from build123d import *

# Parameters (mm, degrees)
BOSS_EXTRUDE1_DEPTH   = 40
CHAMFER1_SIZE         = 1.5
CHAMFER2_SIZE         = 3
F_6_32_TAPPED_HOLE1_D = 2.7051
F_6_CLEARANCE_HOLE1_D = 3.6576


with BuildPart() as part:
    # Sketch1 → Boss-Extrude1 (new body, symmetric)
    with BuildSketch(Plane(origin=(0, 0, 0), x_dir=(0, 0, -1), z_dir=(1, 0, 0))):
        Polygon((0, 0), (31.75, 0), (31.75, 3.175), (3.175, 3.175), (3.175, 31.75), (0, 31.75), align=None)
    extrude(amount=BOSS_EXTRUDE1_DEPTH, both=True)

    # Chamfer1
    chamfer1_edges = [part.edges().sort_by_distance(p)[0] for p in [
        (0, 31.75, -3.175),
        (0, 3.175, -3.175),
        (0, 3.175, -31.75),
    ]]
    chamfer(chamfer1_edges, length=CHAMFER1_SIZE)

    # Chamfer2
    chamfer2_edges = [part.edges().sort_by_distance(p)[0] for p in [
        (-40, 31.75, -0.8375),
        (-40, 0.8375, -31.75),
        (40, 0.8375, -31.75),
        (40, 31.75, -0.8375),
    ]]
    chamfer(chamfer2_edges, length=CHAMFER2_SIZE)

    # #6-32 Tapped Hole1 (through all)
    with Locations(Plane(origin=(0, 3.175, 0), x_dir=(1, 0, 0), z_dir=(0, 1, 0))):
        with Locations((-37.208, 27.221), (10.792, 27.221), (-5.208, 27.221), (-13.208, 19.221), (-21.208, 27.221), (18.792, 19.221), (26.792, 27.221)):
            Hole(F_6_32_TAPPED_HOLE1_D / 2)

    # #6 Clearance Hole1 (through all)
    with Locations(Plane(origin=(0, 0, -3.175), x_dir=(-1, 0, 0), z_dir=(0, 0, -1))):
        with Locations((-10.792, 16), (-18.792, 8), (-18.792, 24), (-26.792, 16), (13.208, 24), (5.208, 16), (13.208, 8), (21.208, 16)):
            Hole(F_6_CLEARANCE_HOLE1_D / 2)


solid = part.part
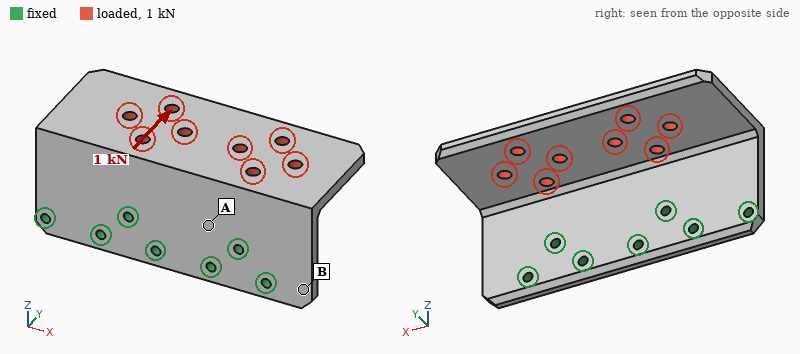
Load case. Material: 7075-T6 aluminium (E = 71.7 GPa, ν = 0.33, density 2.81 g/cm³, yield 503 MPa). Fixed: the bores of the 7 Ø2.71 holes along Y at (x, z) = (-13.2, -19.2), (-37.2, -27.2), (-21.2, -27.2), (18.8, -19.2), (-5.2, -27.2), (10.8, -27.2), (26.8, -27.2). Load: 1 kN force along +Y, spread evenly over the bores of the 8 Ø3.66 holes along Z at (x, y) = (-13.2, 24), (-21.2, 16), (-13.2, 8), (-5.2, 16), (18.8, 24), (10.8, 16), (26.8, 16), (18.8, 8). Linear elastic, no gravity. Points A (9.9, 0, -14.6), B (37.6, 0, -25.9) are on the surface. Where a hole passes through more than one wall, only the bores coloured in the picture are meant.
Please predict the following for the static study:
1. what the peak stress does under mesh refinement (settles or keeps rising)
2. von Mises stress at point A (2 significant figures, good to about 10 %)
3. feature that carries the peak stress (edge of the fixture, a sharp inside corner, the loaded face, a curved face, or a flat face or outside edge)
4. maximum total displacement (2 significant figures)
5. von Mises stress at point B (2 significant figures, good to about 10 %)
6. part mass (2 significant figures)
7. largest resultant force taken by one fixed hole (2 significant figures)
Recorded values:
keeps rising
88 MPa
edge of the fixture
0.42 mm
29 MPa
42 g
880 N
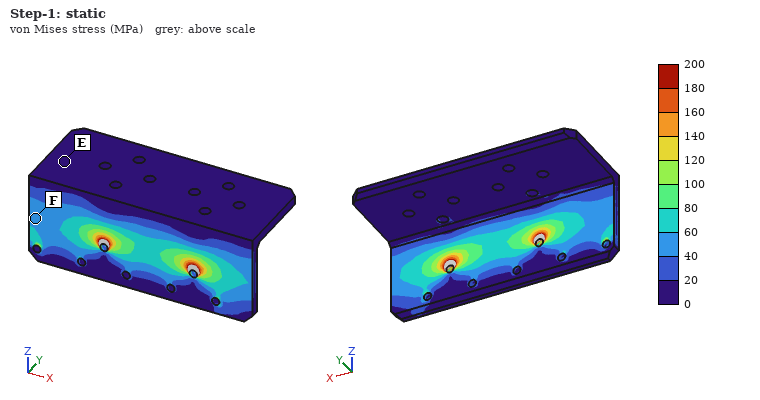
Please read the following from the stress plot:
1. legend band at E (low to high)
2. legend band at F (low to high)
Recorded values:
0 to 20 MPa
40 to 60 MPa
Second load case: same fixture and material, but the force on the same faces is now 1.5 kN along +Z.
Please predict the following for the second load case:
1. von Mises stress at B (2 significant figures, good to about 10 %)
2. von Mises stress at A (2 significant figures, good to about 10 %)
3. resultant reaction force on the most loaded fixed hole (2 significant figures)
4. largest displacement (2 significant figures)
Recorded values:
33 MPa
140 MPa
760 N
1.0 mm
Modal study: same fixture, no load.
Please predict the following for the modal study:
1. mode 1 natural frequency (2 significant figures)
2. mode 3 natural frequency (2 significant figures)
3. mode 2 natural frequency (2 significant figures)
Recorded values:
1500 Hz
3900 Hz
2100 Hz
